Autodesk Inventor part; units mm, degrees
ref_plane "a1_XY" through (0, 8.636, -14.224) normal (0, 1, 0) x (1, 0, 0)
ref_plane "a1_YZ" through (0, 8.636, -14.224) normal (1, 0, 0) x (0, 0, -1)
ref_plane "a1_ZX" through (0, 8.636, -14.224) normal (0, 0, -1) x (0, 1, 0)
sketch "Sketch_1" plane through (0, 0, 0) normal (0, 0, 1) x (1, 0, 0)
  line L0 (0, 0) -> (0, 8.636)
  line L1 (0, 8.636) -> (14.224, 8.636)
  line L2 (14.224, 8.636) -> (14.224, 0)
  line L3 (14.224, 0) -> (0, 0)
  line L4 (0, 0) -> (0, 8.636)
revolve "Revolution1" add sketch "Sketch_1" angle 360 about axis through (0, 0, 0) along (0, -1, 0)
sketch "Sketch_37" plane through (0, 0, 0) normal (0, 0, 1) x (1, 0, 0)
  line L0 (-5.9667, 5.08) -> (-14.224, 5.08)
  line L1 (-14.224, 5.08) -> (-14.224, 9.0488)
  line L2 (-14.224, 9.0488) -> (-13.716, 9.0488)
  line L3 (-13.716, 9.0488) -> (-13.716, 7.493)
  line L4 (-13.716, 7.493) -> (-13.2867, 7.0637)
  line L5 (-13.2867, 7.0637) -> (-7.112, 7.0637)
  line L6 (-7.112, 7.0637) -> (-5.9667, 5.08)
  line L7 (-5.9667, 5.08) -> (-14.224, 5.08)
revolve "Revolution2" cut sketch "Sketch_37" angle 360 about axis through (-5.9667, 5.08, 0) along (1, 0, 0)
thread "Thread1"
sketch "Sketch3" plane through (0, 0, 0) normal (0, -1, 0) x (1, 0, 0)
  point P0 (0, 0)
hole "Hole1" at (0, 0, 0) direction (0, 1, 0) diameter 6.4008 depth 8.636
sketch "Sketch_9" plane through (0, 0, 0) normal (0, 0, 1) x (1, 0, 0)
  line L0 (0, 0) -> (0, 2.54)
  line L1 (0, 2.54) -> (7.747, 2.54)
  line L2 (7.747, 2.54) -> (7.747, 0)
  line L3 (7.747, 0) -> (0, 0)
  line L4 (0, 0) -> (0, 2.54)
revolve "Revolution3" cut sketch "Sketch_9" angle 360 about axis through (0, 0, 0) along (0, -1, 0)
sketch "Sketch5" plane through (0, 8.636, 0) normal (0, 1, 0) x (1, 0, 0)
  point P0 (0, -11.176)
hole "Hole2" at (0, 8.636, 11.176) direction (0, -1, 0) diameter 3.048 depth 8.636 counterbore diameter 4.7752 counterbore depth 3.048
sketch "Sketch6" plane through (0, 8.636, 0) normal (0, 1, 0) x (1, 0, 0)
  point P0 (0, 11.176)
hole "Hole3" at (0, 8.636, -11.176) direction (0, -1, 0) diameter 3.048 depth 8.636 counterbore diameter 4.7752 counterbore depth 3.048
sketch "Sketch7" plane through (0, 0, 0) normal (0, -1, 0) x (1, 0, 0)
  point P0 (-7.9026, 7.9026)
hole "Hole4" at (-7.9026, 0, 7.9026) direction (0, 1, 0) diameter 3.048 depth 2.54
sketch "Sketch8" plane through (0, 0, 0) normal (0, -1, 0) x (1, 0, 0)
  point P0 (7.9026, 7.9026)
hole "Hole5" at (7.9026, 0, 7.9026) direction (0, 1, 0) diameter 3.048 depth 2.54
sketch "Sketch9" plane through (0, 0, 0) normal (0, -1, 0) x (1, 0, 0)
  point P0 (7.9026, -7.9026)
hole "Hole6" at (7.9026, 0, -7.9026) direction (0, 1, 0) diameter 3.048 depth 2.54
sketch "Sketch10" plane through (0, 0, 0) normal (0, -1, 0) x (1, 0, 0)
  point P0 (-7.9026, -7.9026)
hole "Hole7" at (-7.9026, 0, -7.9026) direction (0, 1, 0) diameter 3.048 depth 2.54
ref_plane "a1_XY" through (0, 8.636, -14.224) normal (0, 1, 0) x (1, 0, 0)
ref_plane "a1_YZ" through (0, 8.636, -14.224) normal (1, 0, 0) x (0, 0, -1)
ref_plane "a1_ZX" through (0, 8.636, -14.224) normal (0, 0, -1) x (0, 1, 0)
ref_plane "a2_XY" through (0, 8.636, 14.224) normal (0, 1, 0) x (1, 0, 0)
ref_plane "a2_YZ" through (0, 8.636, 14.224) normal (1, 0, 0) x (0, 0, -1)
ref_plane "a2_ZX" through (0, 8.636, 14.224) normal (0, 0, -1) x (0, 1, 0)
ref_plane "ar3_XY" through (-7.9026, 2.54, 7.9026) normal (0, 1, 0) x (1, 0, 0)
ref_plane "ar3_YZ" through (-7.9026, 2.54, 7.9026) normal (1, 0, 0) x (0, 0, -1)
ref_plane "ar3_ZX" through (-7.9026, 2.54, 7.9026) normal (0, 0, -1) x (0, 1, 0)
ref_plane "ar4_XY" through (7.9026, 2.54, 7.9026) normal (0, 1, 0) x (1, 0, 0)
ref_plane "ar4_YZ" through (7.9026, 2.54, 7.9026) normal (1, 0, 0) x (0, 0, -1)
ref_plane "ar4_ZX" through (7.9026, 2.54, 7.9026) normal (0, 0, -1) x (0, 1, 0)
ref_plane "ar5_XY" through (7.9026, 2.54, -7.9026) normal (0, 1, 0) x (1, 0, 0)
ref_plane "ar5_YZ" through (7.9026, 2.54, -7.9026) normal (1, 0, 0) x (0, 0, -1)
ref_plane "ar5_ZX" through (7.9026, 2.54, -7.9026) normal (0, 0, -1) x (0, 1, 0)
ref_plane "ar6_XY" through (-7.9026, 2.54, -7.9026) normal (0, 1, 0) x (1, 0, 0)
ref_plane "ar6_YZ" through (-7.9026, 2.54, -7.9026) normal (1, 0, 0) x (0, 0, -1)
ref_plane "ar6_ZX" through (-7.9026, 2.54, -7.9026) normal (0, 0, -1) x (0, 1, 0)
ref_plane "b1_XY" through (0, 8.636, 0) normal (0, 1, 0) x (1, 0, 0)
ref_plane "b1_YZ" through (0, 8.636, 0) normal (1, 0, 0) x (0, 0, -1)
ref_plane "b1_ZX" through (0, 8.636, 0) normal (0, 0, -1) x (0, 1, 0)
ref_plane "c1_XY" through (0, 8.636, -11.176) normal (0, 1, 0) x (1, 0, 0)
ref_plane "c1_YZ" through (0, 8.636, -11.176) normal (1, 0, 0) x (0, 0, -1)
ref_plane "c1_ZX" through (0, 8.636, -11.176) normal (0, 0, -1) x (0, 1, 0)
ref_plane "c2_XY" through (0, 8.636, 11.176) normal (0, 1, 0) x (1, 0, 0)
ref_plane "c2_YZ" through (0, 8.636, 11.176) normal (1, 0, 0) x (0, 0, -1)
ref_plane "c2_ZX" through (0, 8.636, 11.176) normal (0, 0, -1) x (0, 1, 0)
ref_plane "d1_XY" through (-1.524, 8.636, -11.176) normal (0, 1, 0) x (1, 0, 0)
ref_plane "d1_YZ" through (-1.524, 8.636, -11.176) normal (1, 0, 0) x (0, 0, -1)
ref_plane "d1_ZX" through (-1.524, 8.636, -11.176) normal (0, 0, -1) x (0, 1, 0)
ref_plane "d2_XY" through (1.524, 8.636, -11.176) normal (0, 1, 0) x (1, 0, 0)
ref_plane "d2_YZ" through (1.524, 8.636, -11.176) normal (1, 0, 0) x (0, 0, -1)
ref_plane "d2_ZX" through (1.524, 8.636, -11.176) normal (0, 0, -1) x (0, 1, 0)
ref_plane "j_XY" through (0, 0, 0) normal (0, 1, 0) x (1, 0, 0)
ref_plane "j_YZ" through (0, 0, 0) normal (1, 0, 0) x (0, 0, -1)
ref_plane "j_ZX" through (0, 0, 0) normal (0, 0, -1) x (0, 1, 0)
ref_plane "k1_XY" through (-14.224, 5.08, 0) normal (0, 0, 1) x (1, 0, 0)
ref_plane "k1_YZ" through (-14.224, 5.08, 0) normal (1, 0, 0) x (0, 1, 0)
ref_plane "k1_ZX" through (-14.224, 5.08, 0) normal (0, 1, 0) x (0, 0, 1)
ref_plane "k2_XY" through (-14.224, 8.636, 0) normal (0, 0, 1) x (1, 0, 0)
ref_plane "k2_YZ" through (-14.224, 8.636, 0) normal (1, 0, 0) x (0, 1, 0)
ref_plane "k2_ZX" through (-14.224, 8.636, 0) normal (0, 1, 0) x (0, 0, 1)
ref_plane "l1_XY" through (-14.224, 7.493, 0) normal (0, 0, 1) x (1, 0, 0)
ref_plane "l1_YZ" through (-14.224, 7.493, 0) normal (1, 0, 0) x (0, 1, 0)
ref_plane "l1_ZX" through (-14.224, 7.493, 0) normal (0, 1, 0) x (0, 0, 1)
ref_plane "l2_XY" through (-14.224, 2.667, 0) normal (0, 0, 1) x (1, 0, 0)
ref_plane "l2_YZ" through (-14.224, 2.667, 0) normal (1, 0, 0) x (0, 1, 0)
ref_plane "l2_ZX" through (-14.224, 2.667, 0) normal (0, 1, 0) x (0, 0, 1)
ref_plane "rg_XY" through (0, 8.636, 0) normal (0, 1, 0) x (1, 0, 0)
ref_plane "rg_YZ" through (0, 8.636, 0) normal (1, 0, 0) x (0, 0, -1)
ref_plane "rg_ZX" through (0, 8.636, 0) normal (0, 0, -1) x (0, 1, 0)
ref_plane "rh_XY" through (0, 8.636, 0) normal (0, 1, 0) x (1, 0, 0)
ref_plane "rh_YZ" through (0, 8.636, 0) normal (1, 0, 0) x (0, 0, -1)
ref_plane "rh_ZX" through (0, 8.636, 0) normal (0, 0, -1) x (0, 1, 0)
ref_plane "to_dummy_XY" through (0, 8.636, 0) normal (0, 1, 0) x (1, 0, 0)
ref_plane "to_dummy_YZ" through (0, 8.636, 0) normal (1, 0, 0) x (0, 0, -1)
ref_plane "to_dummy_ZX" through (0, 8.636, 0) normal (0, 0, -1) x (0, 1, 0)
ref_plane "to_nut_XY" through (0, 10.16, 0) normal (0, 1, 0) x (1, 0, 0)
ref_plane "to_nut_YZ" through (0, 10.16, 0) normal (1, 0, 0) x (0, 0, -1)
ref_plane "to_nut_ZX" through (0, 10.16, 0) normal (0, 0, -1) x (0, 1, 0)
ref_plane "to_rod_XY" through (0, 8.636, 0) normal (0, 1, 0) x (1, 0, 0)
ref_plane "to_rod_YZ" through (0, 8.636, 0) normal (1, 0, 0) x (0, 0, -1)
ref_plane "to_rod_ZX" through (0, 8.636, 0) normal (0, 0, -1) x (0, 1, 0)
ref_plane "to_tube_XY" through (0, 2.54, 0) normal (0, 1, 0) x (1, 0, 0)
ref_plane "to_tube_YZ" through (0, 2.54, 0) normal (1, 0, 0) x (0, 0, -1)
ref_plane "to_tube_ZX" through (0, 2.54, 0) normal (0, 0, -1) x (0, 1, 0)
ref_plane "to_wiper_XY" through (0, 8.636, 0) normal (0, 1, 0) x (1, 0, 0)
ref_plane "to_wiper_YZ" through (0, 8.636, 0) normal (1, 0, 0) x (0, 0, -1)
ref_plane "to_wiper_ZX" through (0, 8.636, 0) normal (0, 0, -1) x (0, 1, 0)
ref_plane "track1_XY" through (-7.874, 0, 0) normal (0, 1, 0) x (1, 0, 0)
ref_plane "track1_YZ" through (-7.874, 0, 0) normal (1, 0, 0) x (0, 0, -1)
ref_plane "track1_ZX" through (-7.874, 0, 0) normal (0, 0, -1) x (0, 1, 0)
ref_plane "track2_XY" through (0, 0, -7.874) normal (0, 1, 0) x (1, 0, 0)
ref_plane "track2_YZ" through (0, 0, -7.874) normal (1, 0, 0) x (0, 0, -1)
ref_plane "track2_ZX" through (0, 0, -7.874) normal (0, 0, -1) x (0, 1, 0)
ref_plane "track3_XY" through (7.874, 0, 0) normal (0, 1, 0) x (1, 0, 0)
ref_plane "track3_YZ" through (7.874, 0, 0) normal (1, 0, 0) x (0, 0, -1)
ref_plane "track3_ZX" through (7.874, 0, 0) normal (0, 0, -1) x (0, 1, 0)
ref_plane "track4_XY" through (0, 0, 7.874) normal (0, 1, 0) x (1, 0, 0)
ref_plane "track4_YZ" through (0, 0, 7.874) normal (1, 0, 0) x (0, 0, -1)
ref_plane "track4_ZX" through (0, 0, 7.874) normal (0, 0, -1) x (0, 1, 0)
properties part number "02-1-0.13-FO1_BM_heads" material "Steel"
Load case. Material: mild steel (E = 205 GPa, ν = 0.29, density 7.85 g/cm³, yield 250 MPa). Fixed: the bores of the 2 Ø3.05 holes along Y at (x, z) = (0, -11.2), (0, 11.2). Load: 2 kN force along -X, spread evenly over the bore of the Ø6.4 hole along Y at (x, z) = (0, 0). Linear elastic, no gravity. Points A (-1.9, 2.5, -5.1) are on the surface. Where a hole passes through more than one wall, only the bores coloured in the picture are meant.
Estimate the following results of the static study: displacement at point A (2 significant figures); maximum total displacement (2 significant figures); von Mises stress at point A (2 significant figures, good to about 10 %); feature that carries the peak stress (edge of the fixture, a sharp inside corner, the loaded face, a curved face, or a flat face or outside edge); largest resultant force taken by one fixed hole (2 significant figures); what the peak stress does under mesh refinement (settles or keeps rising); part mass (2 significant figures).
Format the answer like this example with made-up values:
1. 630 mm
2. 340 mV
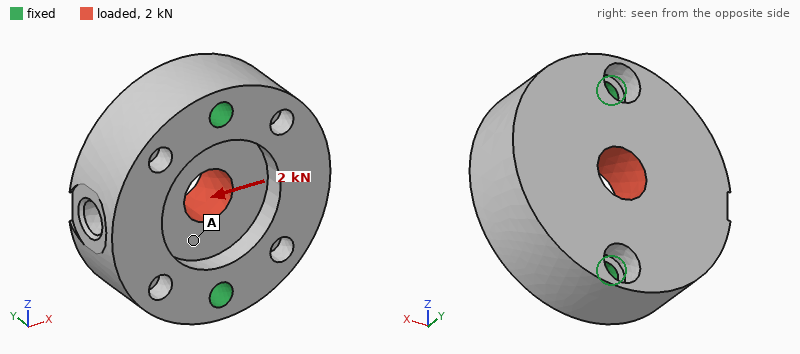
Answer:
1. 0.86 µm
2. 3.4 µm
3. 15 MPa
4. edge of the fixture
5. 1.0 kN
6. keeps rising
7. 35 g
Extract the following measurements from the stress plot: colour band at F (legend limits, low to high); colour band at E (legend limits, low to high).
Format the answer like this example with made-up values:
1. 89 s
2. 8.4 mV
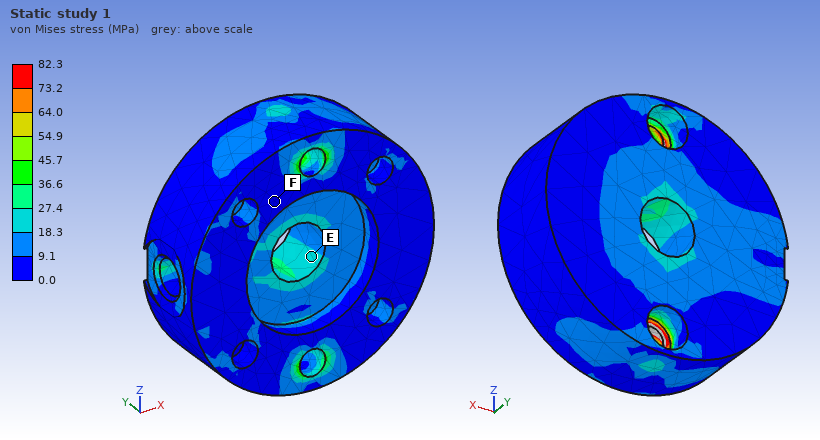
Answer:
1. 0.0 to 9.1 MPa
2. 18.3 to 27.4 MPa
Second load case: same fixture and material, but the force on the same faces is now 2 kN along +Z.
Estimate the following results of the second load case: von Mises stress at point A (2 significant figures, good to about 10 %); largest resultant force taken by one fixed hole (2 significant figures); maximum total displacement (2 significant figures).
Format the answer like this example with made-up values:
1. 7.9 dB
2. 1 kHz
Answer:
1. 24 MPa
2. 1.0 kN
3. 1.1 µm
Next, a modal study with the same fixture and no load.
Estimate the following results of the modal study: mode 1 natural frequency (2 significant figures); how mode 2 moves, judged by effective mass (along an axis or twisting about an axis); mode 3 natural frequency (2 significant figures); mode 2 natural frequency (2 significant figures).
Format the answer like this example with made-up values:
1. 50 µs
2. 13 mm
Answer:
1. 17 kHz
2. along Y
3. 41 kHz
4. 25 kHz
